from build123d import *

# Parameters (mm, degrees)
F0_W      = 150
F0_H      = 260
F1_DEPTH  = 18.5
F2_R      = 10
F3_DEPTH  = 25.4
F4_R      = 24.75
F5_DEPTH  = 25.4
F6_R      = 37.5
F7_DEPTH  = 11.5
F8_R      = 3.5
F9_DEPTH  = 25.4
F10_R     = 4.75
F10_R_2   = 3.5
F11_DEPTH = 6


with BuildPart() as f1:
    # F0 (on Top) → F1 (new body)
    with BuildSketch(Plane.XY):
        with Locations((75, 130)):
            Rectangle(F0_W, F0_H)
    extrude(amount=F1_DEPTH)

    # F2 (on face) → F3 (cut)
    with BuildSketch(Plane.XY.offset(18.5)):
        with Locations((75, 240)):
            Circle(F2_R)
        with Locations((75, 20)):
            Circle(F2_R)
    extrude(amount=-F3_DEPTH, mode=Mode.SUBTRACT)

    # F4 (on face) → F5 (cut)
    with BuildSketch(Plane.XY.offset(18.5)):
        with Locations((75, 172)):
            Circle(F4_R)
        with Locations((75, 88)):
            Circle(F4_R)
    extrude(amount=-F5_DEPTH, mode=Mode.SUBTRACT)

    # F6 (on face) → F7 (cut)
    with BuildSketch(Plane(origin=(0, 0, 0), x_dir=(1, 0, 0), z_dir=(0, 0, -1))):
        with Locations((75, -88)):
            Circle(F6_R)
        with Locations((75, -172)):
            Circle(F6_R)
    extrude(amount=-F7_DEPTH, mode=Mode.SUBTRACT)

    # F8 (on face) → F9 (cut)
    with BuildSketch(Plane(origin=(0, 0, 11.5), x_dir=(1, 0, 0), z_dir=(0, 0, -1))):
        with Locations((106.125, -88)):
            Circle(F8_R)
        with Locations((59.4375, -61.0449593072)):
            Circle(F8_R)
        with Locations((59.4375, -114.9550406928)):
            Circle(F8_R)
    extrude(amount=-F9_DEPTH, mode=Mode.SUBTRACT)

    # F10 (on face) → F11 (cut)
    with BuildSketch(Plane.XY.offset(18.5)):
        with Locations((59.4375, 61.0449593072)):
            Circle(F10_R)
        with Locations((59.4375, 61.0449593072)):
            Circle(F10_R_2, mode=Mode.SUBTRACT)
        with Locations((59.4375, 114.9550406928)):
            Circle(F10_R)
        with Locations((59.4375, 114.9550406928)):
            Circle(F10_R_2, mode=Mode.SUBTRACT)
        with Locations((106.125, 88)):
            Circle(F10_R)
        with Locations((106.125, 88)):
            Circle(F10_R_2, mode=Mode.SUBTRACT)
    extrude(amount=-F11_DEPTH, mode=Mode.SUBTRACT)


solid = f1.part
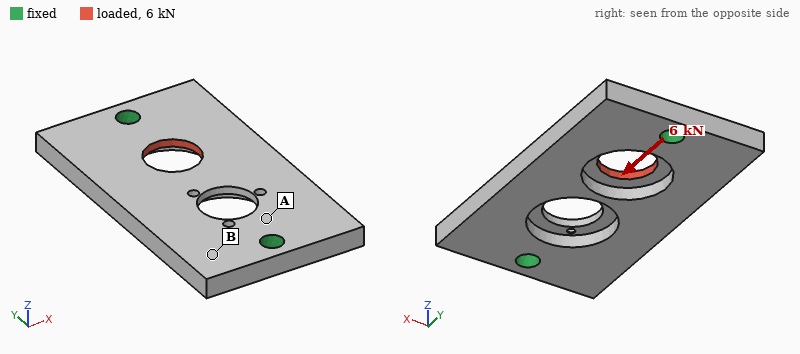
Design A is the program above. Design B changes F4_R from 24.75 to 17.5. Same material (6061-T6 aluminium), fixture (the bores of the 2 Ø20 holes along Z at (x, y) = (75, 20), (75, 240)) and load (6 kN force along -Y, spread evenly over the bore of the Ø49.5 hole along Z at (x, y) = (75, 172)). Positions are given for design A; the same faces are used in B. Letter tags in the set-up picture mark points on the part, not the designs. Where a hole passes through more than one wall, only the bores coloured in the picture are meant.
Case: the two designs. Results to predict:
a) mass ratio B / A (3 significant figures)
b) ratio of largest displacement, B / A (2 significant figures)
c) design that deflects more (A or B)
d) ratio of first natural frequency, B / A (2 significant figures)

1.02
0.87
A
1.0
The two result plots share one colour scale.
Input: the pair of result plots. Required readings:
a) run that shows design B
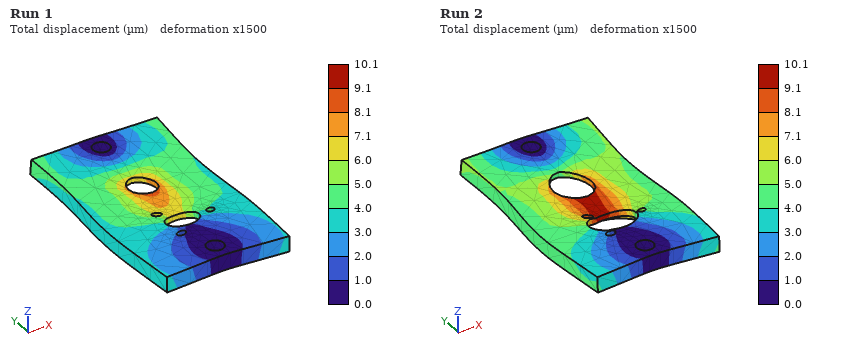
Run 1
